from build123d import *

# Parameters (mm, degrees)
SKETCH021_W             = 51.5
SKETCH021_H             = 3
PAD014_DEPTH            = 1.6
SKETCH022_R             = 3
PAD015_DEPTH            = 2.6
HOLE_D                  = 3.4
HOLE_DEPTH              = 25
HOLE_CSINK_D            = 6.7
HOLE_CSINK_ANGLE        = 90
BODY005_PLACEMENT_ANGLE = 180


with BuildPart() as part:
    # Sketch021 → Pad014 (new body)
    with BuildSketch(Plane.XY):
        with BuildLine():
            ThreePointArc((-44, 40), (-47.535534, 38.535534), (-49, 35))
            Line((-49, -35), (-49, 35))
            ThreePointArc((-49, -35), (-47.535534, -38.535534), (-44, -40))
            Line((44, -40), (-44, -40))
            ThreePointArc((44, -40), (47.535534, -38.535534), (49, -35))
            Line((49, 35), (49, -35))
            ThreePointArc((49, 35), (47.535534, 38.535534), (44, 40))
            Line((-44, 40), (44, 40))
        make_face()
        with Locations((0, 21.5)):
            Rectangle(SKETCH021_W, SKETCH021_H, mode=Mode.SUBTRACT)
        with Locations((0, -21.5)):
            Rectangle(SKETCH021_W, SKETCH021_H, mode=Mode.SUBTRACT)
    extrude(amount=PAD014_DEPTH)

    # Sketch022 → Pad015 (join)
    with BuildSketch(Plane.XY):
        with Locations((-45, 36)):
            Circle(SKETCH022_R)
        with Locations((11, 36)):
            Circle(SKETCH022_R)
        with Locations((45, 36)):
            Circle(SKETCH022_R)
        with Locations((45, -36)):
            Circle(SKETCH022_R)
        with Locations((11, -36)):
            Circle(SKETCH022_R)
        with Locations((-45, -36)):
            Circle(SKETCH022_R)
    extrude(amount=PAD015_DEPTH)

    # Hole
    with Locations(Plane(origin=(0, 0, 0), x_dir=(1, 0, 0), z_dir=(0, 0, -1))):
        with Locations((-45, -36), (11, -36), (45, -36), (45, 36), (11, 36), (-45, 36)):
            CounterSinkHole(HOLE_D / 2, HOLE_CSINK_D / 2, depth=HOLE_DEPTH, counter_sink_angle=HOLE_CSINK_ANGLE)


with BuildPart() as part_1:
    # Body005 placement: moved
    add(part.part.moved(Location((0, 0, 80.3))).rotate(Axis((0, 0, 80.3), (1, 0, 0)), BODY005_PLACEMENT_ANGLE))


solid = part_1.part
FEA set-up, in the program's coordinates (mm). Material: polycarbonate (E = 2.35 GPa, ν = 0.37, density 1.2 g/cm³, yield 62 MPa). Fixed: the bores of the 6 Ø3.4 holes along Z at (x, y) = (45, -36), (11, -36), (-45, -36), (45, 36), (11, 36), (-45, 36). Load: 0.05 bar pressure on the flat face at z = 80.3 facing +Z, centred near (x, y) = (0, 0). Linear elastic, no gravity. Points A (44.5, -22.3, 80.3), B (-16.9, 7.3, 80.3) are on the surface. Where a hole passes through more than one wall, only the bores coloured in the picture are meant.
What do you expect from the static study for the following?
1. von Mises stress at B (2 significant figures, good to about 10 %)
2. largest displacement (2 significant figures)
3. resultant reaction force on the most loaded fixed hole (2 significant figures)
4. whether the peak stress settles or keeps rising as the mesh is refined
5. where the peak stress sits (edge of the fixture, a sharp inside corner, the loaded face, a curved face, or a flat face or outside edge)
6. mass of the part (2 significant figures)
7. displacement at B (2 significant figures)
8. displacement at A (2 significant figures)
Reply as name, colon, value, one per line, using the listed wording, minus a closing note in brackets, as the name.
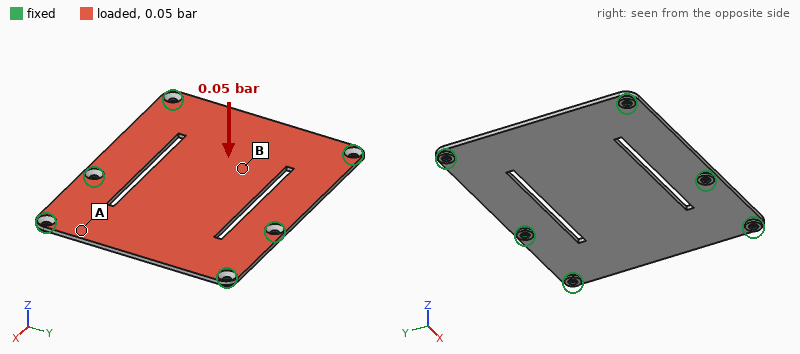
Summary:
von Mises stress at B: 2.8 MPa
largest displacement: 1.3 mm
resultant reaction force on the most loaded fixed hole: 18 N
whether the peak stress settles or keeps rising as the mesh is refined: keeps rising
where the peak stress sits: edge of the fixture
mass of the part: 14 g
displacement at B: 1.2 mm
displacement at A: 0.23 mm
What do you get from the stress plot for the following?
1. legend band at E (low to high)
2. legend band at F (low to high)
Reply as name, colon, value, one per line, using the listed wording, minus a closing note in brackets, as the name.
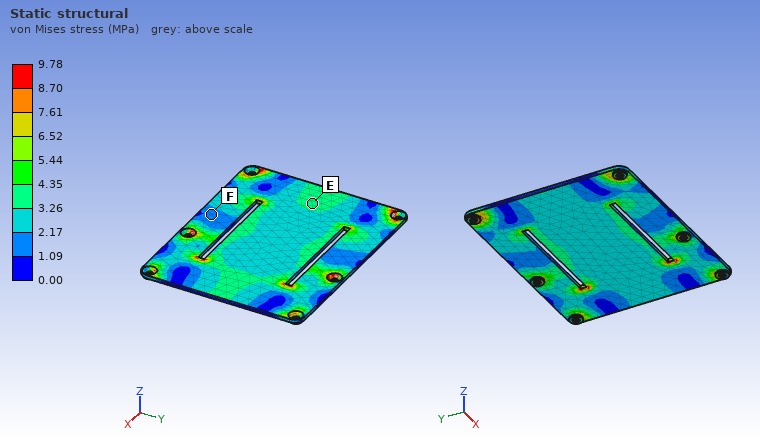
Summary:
legend band at E: 3.26 to 4.35 MPa
legend band at F: 1.09 to 2.17 MPa
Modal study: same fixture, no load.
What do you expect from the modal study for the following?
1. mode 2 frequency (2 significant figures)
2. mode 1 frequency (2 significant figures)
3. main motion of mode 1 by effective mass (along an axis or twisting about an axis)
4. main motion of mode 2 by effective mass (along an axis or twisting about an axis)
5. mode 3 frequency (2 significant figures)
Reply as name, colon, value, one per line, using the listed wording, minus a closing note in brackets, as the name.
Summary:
mode 2 frequency: 440 Hz
mode 1 frequency: 270 Hz
main motion of mode 1 by effective mass: along Z
main motion of mode 2 by effective mass: twisting about Y
mode 3 frequency: 570 Hz
